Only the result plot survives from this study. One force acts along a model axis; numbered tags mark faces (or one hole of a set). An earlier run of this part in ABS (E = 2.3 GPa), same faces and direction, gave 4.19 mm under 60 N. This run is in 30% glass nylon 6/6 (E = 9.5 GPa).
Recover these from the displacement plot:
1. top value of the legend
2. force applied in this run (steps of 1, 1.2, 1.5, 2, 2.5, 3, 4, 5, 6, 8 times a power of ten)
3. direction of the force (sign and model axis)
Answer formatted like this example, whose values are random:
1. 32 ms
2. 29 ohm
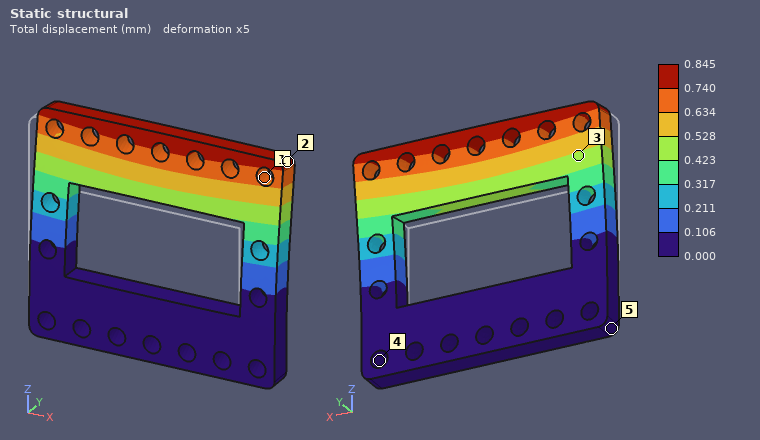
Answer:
1. 0.845 mm
2. 50 N
3. +Y
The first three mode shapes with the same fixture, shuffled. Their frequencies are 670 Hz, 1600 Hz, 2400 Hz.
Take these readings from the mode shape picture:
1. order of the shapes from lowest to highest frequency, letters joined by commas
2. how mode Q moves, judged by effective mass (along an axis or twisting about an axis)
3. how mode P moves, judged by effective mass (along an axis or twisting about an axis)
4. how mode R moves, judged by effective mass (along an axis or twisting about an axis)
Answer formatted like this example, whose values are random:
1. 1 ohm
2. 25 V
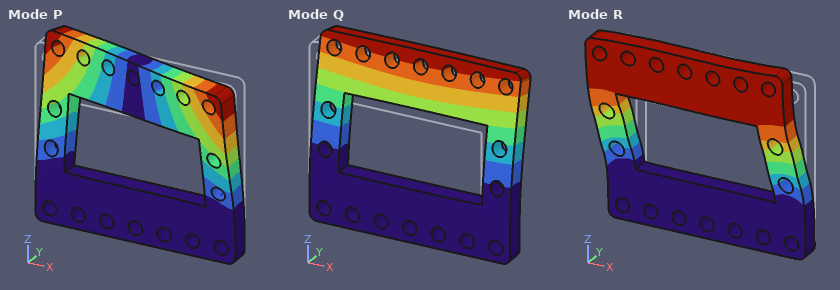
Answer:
1. Q, P, R
2. along Y
3. twisting about Z
4. along X
